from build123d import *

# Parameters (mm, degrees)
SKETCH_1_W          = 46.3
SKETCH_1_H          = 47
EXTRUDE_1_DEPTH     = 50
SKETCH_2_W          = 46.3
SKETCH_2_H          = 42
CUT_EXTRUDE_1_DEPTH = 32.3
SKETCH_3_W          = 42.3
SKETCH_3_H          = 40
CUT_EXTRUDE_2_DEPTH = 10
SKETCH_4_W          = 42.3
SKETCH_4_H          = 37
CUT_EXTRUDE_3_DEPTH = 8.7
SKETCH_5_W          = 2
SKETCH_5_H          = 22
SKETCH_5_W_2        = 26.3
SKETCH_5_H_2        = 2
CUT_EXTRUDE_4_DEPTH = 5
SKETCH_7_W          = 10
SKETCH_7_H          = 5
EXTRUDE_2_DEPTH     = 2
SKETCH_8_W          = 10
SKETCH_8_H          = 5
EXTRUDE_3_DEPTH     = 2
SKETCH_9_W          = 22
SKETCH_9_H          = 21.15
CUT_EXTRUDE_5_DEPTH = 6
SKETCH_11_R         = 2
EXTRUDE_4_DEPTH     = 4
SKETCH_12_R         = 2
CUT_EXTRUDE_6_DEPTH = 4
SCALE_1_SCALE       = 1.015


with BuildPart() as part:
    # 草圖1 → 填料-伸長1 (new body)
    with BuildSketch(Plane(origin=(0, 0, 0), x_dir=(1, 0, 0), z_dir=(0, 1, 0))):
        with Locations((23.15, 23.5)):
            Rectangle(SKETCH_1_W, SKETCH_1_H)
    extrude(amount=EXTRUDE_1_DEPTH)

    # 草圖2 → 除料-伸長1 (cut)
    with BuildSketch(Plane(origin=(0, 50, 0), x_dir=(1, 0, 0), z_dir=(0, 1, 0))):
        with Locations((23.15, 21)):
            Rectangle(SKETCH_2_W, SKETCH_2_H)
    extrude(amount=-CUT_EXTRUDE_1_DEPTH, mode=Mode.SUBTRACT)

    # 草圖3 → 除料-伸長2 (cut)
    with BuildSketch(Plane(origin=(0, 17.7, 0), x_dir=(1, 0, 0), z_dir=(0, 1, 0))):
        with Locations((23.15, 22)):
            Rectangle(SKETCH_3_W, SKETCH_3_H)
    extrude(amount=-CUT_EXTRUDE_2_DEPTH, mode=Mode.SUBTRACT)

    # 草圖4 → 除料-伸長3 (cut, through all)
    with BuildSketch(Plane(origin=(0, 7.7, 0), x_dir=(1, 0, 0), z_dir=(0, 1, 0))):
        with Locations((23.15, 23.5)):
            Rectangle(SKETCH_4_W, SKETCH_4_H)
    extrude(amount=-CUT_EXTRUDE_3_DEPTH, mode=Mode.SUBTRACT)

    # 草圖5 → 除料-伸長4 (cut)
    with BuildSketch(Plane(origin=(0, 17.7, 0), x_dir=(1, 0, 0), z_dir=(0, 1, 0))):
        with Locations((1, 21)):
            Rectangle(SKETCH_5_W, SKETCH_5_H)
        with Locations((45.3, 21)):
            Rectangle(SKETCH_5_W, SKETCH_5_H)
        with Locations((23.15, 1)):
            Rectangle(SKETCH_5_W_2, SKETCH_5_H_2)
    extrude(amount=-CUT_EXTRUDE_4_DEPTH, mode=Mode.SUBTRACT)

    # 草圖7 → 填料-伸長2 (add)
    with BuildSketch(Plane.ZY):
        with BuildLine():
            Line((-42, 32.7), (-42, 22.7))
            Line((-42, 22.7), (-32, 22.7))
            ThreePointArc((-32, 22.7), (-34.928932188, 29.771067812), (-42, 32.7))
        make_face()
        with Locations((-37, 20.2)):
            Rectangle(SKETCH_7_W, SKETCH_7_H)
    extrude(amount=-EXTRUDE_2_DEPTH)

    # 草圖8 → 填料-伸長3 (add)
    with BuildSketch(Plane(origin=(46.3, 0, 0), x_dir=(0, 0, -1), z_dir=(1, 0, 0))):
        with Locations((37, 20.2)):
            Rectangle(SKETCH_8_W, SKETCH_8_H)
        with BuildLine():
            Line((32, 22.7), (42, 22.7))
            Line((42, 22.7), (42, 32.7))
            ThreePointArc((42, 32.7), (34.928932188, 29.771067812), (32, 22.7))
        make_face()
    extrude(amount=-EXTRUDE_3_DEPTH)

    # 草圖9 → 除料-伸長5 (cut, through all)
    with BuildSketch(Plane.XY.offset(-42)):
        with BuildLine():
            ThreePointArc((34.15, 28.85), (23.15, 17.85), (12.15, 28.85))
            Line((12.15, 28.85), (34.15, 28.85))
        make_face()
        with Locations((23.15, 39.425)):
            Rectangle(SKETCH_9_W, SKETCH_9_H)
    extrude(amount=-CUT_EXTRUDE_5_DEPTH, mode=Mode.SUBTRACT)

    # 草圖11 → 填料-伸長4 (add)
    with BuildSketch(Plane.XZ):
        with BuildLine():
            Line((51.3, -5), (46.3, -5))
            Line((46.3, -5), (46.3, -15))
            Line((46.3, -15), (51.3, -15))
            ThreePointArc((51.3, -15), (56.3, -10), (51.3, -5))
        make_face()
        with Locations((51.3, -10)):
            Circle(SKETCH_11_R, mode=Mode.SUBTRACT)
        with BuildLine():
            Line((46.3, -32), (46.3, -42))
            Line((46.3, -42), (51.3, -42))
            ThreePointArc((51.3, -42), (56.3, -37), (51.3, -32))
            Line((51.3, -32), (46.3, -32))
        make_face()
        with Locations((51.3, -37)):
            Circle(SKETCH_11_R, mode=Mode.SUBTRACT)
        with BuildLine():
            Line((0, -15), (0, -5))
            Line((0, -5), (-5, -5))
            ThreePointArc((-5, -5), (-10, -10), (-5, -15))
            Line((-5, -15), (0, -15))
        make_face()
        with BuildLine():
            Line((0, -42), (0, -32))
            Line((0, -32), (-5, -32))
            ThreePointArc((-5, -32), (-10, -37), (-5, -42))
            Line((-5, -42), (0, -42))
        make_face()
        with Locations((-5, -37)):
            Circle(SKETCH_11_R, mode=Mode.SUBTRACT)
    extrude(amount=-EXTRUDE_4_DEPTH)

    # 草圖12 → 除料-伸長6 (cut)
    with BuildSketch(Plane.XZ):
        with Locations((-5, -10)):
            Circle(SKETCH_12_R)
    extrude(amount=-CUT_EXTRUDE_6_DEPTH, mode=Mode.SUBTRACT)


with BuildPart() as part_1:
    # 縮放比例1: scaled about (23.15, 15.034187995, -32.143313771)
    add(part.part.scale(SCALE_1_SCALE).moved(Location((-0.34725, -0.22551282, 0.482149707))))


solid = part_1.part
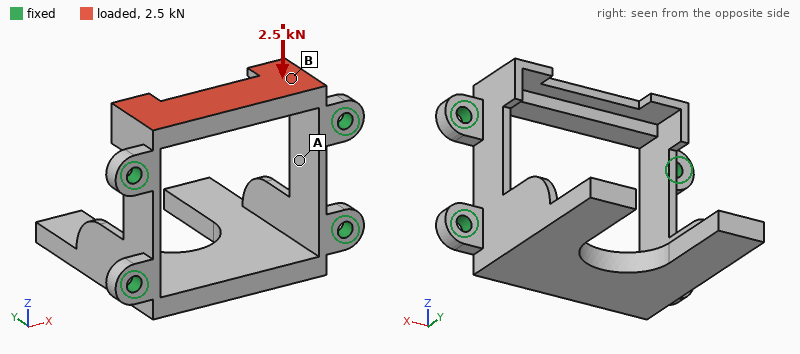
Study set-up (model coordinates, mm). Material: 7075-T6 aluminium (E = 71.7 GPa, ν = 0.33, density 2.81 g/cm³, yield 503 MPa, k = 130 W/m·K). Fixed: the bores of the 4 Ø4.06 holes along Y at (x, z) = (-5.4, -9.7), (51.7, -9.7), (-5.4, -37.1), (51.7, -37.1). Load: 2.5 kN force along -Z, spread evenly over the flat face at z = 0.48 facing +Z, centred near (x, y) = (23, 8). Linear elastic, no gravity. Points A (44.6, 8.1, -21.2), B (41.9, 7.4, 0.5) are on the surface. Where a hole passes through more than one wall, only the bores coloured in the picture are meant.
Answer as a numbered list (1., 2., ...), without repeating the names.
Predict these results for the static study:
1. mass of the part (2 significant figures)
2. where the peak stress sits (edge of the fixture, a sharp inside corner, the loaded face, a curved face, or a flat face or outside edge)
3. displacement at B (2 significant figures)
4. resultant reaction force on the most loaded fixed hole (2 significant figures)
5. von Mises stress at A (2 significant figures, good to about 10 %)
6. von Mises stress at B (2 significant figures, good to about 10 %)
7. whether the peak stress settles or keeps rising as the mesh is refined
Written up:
1. 43 g
2. a sharp inside corner
3. 0.078 mm
4. 1.5 kN
5. 27 MPa
6. 61 MPa
7. keeps rising
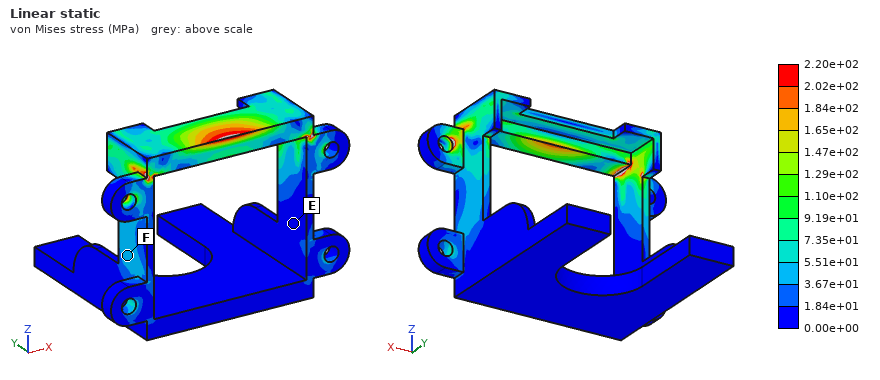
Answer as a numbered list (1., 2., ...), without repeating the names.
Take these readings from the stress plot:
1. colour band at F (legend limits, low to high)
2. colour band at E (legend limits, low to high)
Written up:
1. 3.67e+01 to 5.51e+01 MPa
2. 0.00e+00 to 1.84e+01 MPa
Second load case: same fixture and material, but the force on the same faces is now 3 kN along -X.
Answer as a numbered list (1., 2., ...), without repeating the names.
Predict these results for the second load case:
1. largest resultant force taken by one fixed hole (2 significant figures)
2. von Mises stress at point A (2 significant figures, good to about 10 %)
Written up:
1. 1.6 kN
2. 16 MPa
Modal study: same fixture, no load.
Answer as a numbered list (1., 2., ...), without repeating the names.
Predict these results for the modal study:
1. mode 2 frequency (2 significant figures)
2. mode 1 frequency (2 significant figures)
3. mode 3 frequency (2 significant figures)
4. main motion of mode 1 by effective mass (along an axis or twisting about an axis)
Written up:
1. 3300 Hz
2. 2700 Hz
3. 6100 Hz
4. along Z
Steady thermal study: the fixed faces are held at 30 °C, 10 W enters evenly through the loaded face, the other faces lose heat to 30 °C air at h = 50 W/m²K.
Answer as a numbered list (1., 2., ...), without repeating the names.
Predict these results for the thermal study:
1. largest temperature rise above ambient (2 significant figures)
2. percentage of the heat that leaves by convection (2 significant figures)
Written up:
1. 17 K
2. 14 %
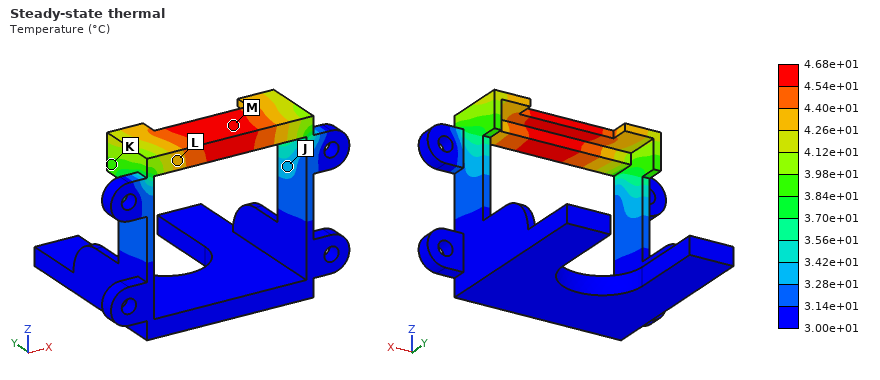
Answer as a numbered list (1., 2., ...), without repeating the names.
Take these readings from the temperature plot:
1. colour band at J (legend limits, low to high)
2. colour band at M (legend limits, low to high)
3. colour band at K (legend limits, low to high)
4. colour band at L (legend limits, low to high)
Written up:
1. 3.28e+01 to 3.42e+01 °C
2. 4.54e+01 to 4.68e+01 °C
3. 3.84e+01 to 3.98e+01 °C
4. 4.26e+01 to 4.40e+01 °C
